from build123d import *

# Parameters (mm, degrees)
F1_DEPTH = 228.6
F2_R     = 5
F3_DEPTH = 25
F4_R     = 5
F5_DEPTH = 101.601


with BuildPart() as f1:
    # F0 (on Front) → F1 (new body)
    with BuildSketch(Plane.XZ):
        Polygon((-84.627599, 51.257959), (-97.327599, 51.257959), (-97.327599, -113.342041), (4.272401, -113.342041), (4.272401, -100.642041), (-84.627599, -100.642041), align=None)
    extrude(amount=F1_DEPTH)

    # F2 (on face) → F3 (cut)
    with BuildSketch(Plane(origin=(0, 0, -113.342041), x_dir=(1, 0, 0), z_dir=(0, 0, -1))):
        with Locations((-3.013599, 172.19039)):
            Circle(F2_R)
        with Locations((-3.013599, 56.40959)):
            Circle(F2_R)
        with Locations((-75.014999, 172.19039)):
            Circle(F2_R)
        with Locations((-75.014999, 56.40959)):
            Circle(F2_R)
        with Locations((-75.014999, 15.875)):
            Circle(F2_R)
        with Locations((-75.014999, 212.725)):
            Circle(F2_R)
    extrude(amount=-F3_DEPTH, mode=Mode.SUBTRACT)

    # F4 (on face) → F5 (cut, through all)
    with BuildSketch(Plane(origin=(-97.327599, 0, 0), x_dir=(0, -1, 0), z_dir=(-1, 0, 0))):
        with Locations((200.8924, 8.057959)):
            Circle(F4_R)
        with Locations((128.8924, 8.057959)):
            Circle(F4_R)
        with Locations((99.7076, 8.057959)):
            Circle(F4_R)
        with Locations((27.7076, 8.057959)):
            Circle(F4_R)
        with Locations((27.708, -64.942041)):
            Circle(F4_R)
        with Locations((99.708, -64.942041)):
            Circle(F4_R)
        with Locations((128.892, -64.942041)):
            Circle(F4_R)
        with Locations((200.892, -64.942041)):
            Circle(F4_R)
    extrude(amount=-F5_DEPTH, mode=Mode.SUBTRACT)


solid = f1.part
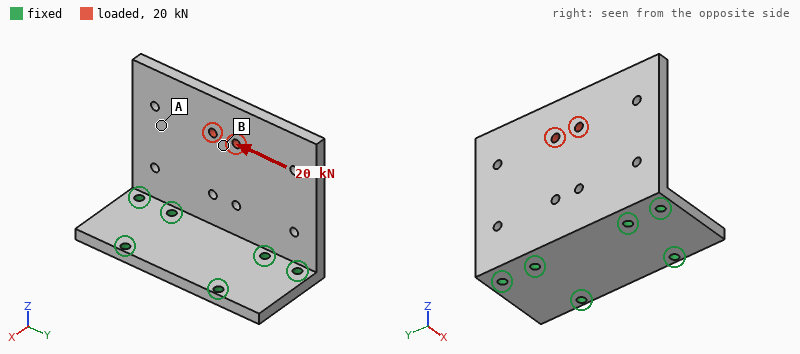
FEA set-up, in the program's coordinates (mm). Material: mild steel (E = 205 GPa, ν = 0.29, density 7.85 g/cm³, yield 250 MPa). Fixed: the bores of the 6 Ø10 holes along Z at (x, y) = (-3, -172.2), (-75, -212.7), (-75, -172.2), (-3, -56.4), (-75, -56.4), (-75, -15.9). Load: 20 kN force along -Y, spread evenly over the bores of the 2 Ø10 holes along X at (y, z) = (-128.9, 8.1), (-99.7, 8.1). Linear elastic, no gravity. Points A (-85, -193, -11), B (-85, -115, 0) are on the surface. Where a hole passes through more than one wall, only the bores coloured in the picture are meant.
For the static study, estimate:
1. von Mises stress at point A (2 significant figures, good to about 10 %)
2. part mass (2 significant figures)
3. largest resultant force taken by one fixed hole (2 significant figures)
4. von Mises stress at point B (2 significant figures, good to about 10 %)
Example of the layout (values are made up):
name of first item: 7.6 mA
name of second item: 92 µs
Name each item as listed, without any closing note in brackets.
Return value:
von Mises stress at point A: 10 MPa
part mass: 5.7 kg
largest resultant force taken by one fixed hole: 9.7 kN
von Mises stress at point B: 31 MPa
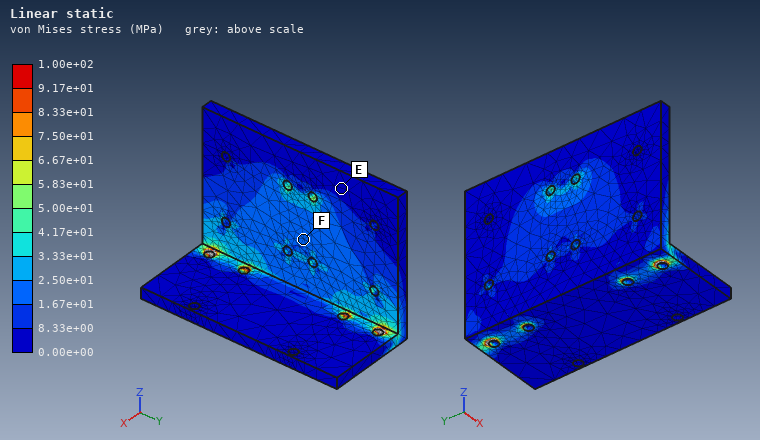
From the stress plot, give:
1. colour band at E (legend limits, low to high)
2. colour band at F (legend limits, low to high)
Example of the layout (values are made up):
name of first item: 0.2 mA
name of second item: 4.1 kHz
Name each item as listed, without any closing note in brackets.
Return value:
colour band at E: 0.00e+00 to 8.33e+00 MPa
colour band at F: 1.67e+01 to 2.50e+01 MPa
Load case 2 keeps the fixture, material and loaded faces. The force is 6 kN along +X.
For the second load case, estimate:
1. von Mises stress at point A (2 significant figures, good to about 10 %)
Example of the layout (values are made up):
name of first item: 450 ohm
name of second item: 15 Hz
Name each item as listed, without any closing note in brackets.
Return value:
von Mises stress at point A: 25 MPa
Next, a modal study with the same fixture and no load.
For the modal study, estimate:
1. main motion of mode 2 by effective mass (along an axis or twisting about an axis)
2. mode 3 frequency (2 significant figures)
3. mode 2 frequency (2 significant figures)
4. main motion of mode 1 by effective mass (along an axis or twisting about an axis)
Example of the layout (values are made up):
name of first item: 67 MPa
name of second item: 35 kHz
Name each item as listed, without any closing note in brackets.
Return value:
main motion of mode 2 by effective mass: twisting about Z
mode 3 frequency: 1800 Hz
mode 2 frequency: 730 Hz
main motion of mode 1 by effective mass: along X
